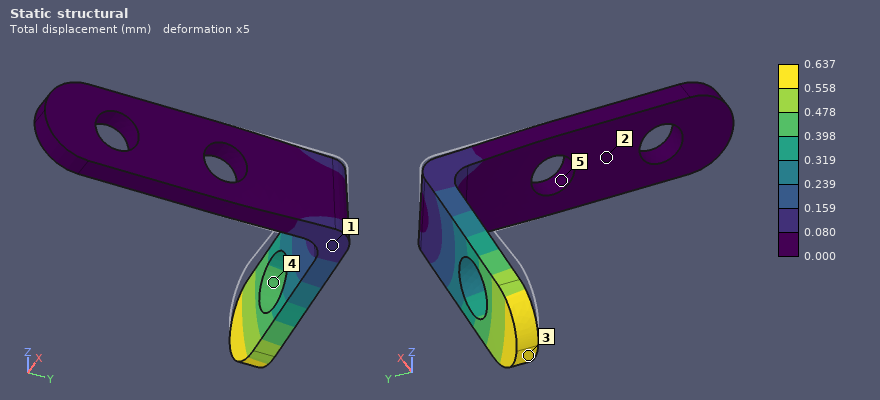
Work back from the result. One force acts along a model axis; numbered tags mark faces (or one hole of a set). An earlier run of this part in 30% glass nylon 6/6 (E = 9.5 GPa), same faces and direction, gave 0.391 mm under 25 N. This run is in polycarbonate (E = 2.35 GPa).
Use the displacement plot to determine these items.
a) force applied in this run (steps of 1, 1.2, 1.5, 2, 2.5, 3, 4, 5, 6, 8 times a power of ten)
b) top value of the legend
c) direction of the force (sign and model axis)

10 N
0.637 mm
-Z
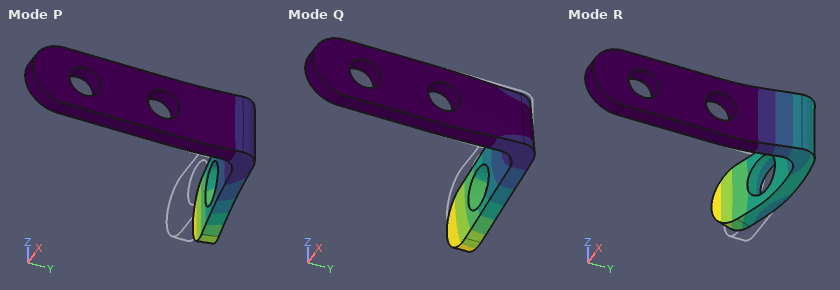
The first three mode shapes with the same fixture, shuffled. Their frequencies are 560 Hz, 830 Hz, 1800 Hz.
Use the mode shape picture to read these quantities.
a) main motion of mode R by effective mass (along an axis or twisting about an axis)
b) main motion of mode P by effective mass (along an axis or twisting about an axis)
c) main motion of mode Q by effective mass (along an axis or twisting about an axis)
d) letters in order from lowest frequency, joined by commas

along X
along Y
along Z
P, Q, R
